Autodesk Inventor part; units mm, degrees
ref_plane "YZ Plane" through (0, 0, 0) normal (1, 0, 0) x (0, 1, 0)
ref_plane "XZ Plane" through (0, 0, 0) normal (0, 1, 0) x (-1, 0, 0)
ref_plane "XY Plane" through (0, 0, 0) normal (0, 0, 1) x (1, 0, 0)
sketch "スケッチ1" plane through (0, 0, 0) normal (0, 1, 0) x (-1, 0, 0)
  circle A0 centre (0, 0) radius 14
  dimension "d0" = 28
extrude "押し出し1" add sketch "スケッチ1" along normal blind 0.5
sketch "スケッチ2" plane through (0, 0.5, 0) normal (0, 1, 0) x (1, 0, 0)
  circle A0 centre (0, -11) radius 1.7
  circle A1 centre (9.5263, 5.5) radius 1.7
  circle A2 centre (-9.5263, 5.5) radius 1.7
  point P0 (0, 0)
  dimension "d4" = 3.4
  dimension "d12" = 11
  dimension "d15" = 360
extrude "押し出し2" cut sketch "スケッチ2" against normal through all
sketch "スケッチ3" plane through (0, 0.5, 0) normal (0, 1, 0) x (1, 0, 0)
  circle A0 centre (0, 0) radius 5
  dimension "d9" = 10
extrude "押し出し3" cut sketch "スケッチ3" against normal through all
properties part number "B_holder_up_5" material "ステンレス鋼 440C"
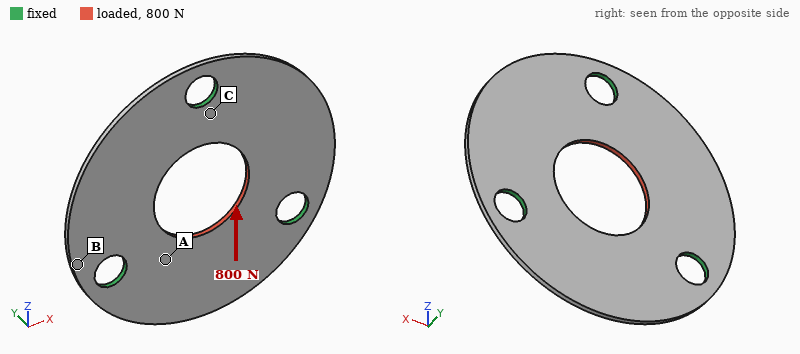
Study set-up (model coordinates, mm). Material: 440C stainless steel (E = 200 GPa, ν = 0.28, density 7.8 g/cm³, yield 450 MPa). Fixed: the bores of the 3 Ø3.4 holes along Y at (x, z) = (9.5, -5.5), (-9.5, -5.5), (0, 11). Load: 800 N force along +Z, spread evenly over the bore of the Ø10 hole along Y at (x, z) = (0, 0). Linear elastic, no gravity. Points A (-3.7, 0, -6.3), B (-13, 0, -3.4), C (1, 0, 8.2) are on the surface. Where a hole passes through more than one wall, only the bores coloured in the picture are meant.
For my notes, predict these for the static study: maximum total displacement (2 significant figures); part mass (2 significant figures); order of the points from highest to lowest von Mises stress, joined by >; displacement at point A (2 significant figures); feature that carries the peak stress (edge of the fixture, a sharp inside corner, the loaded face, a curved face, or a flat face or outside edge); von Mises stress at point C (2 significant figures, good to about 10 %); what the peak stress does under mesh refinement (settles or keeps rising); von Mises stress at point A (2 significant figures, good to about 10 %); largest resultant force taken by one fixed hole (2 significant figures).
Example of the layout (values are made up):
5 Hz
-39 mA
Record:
4.4 µm
2.0 g
C > A > B
3.0 µm
edge of the fixture
82 MPa
keeps rising
48 MPa
280 N
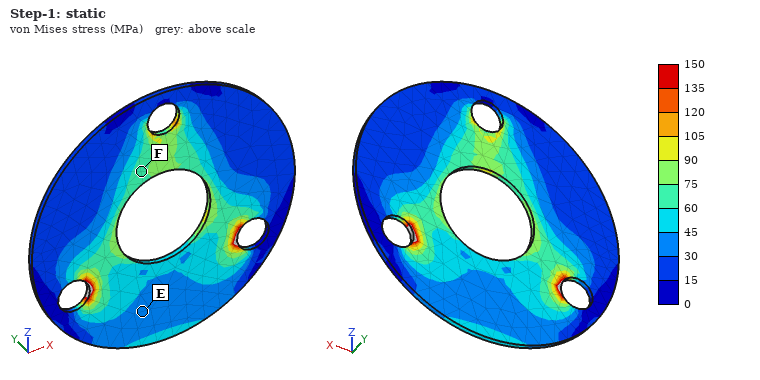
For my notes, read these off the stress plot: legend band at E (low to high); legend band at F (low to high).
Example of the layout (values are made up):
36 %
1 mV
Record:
30 to 45 MPa
60 to 75 MPa
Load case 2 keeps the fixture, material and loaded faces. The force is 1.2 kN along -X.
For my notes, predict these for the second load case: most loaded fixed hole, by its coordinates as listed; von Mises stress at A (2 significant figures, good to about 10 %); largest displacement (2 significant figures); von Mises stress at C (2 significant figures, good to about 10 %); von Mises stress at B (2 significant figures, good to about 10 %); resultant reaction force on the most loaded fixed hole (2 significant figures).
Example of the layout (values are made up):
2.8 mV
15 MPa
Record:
(0, 11)
78 MPa
5.9 µm
110 MPa
20 MPa
440 N
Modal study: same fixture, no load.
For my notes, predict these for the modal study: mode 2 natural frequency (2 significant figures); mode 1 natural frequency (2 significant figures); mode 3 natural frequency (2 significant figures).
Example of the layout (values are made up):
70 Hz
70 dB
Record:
5800 Hz
5800 Hz
5900 Hz
